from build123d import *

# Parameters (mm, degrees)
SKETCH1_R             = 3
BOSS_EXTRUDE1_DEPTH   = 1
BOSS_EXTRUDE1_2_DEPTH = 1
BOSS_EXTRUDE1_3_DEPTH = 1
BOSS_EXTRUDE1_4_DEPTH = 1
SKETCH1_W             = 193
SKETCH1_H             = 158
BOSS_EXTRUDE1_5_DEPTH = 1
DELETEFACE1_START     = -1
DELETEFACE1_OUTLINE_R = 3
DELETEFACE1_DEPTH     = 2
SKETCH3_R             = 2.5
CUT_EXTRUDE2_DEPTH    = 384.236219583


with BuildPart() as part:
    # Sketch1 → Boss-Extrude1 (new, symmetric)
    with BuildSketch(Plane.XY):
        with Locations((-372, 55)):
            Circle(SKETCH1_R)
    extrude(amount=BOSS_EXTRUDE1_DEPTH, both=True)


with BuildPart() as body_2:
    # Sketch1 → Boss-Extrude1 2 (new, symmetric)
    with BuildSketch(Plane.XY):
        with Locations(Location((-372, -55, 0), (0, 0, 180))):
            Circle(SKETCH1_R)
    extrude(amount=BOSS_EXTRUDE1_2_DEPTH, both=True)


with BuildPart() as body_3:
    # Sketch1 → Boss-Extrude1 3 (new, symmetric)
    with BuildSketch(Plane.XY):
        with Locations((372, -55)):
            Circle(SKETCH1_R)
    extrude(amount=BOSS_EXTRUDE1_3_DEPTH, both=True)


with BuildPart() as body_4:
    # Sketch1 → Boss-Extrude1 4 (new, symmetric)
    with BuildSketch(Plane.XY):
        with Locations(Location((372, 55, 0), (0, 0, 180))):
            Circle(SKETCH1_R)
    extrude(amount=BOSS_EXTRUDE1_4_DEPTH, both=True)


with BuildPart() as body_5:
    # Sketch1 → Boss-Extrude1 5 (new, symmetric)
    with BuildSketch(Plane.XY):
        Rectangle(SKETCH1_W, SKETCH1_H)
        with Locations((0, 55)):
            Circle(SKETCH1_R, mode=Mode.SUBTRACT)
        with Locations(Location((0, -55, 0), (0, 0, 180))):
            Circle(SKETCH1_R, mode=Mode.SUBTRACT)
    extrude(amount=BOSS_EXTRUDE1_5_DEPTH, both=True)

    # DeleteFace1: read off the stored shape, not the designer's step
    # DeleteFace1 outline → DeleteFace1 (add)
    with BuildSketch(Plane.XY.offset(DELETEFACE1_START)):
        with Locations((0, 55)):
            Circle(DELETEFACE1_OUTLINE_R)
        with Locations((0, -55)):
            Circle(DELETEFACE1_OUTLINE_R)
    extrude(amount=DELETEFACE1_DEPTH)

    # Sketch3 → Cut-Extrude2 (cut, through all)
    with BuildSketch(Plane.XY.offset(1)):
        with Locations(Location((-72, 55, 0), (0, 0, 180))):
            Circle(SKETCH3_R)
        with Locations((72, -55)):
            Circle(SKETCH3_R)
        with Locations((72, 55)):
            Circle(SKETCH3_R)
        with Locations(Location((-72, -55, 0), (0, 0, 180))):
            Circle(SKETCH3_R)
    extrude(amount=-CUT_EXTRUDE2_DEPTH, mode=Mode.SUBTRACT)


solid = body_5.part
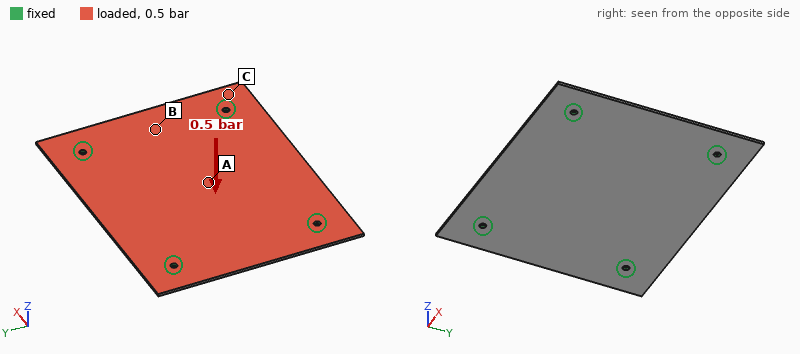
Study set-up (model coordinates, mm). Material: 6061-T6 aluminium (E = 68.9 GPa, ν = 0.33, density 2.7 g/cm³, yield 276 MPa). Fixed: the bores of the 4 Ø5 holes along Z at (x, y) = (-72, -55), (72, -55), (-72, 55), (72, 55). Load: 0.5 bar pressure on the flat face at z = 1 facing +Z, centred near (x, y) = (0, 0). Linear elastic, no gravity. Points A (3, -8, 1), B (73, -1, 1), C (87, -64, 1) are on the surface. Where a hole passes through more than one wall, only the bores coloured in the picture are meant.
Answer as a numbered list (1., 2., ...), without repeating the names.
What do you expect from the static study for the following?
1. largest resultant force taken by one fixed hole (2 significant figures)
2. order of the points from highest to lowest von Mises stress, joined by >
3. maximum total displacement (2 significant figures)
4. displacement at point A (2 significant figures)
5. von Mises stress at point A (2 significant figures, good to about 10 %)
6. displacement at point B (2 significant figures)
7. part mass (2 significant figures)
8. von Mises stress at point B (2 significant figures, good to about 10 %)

1. 380 N
2. A > B > C
3. 1.9 mm
4. 1.9 mm
5. 65 MPa
6. 0.60 mm
7. 160 g
8. 51 MPa
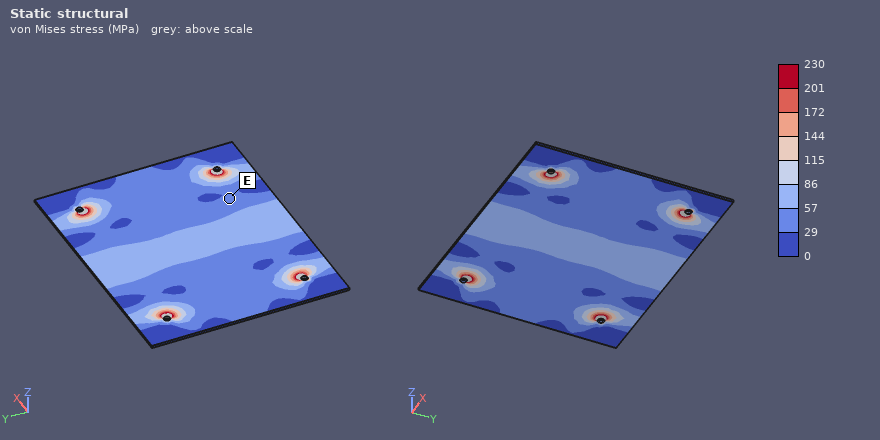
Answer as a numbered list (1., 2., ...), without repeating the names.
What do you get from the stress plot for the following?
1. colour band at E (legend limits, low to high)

1. 29 to 57 MPa
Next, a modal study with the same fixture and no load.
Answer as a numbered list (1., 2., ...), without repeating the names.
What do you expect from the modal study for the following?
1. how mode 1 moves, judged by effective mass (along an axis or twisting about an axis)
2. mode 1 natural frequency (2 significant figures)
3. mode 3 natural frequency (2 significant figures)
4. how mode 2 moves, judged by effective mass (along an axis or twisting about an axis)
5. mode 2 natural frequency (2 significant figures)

1. along Z
2. 410 Hz
3. 710 Hz
4. twisting about X
5. 560 Hz
